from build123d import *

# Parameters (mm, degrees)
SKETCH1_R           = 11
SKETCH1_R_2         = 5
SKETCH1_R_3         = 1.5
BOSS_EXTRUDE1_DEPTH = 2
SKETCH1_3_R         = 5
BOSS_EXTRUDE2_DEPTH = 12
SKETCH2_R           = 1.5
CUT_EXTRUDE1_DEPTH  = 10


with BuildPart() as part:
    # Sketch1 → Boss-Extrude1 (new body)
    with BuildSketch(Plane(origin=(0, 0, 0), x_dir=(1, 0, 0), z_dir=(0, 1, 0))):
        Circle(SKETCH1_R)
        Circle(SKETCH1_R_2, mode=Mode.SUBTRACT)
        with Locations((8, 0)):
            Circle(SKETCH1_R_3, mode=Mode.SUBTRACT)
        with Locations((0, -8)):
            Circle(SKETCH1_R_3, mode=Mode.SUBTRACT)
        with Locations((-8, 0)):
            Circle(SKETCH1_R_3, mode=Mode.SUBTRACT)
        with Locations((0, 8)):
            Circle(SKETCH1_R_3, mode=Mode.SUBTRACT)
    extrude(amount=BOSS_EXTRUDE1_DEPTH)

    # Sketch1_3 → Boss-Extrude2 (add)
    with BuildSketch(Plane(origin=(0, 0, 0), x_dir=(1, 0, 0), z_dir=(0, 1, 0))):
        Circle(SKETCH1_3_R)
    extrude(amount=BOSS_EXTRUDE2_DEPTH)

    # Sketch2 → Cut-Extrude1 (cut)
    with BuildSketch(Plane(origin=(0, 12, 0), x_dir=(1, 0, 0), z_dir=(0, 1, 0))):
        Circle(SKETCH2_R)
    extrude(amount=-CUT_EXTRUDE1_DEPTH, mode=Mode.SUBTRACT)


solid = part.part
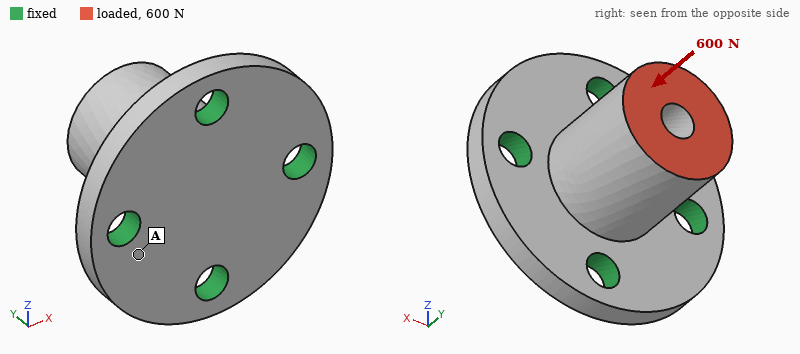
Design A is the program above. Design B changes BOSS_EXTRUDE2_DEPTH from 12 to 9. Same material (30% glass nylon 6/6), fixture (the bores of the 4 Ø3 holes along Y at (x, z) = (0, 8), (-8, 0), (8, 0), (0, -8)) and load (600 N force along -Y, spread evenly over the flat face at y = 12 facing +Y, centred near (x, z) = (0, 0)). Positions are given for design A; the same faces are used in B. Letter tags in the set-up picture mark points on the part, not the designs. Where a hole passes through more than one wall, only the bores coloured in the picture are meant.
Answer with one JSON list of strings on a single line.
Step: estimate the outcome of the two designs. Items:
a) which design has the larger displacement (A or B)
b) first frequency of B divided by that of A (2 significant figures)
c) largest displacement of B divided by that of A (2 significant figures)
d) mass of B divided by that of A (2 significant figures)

["A", "1.5", "0.91", "0.85"]
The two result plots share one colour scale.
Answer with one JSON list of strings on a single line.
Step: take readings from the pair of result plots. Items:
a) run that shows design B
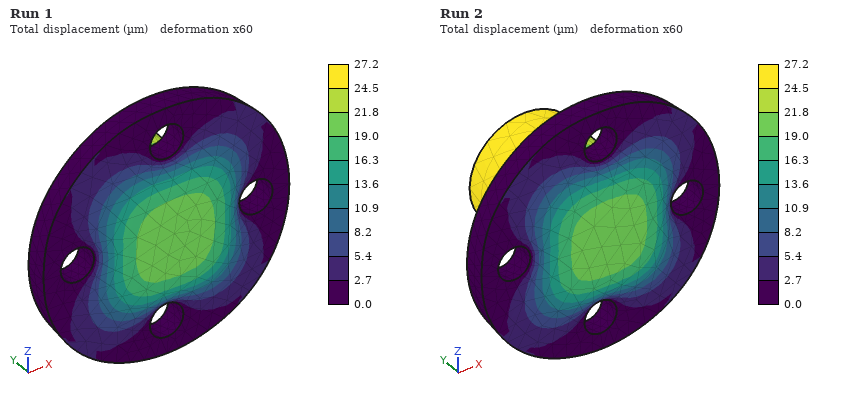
["Run 1"]
